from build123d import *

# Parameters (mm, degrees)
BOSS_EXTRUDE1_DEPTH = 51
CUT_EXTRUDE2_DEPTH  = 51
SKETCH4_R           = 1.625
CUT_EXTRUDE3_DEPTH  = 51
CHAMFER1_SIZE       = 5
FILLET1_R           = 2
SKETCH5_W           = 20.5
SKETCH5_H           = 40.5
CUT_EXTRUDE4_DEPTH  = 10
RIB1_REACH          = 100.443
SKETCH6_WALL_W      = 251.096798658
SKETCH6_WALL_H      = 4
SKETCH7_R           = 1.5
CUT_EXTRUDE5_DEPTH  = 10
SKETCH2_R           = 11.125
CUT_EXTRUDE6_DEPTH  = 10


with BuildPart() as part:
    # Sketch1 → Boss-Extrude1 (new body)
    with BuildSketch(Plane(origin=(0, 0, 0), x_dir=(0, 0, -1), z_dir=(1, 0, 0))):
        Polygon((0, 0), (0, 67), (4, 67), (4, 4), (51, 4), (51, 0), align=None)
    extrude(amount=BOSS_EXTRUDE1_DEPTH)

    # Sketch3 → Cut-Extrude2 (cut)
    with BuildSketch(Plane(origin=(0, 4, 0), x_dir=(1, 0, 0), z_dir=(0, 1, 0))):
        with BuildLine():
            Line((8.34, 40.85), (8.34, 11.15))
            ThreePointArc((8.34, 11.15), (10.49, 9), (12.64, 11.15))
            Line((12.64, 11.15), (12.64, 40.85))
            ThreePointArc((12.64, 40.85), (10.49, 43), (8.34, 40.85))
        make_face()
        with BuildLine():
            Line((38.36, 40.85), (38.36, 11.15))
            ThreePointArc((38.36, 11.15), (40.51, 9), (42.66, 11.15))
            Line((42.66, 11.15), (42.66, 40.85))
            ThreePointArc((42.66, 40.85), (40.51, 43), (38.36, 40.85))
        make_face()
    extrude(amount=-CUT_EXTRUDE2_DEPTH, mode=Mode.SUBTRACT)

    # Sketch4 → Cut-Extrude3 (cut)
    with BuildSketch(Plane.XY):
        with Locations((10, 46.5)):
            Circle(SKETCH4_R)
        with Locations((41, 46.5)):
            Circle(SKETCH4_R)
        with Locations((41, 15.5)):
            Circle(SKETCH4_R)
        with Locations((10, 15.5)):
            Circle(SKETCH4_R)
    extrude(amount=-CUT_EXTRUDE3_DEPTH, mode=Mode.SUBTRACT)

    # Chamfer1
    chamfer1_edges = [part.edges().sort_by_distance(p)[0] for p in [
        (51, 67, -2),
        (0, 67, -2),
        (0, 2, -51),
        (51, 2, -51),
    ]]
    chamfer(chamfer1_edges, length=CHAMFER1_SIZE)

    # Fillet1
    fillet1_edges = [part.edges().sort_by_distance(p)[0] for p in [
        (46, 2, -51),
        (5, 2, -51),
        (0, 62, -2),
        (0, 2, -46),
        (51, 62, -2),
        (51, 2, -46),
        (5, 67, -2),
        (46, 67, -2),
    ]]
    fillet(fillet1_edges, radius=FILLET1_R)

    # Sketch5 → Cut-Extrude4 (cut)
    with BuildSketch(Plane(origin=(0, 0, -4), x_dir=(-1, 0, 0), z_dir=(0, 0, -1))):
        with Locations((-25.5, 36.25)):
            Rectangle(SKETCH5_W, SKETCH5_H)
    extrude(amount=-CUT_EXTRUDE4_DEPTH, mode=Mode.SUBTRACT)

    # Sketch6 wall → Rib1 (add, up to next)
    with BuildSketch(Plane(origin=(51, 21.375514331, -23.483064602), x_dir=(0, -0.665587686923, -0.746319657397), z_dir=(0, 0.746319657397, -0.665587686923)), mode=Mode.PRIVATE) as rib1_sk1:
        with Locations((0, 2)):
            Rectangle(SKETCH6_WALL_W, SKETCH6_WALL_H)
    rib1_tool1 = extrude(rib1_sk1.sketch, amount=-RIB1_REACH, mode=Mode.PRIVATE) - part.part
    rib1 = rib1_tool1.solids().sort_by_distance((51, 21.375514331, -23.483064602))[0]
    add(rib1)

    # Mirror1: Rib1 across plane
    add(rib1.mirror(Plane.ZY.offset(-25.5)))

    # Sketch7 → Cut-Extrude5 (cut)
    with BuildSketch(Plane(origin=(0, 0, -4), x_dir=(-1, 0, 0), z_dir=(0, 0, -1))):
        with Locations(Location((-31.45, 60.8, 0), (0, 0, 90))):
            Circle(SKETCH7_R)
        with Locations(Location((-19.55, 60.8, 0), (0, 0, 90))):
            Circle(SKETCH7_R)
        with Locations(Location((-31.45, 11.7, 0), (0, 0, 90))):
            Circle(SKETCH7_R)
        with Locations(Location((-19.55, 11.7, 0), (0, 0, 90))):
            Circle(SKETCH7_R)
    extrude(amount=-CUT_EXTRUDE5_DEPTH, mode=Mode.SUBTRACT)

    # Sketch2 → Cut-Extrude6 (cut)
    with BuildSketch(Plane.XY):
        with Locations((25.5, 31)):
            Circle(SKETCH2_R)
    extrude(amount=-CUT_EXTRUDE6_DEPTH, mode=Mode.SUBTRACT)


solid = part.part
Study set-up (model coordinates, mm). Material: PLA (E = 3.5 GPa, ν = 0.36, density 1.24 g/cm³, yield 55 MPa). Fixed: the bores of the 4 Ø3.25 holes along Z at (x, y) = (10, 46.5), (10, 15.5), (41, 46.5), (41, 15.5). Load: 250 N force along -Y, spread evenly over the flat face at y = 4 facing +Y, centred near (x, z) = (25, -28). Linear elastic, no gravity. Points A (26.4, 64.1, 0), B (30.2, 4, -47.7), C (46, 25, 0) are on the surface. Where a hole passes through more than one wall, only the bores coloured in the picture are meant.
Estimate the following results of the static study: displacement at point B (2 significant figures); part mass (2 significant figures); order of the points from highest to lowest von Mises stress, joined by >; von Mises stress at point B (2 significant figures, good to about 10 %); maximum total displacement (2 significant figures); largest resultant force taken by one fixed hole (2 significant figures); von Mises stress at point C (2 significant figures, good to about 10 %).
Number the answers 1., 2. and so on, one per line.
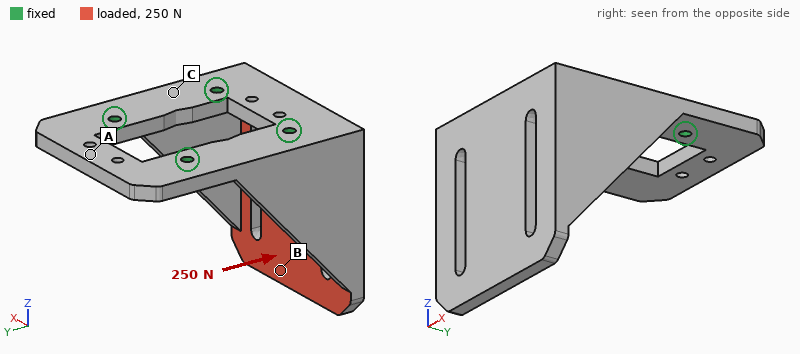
1. 0.92 mm
2. 29 g
3. B > C > A
4. 10 MPa
5. 1.0 mm
6. 140 N
7. 5.1 MPa
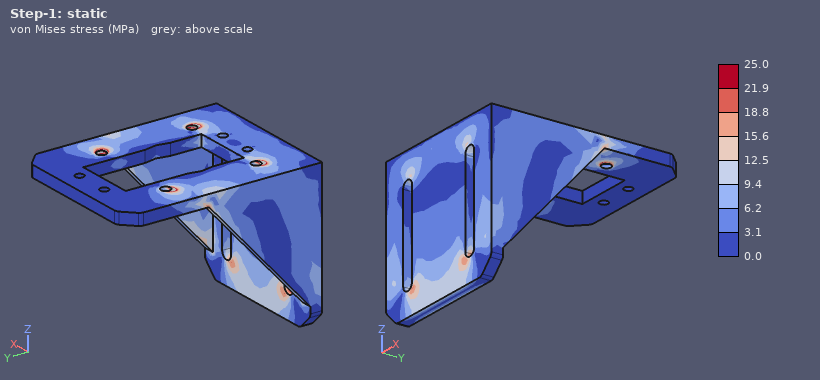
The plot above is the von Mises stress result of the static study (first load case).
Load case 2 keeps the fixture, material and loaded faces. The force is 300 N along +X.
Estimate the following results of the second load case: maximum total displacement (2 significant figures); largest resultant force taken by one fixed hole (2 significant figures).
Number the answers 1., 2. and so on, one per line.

1. 0.68 mm
2. 310 N
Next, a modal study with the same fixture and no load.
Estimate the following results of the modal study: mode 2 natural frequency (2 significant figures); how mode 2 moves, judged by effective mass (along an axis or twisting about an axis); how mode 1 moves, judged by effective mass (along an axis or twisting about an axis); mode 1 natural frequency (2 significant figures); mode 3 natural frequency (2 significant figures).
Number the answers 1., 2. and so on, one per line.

1. 1100 Hz
2. along X
3. along Y
4. 940 Hz
5. 2000 Hz
